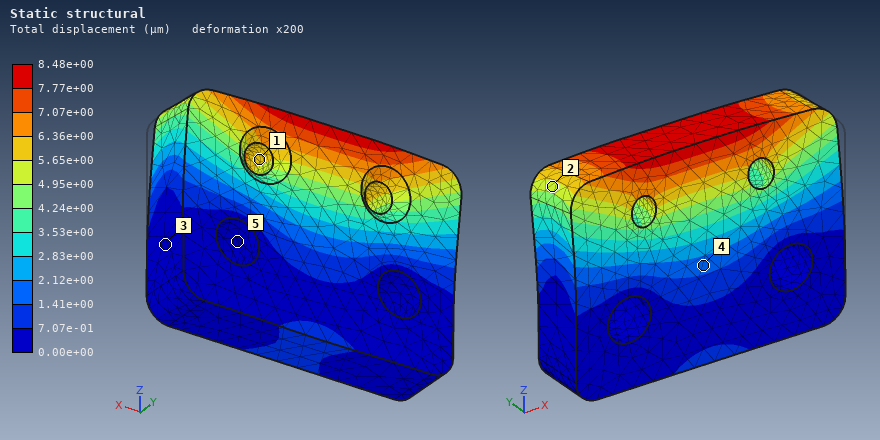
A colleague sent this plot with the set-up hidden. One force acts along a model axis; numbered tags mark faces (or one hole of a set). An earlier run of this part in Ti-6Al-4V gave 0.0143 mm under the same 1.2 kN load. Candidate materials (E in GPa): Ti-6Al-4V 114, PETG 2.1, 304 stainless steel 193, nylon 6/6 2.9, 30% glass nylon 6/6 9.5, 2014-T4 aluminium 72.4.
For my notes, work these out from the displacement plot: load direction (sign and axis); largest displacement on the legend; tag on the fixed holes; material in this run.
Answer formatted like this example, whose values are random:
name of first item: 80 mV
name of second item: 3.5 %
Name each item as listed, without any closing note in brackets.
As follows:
load direction: +Y
largest displacement on the legend: 8.48e+00 µm
tag on the fixed holes: 5
material in this run: 304 stainless steel
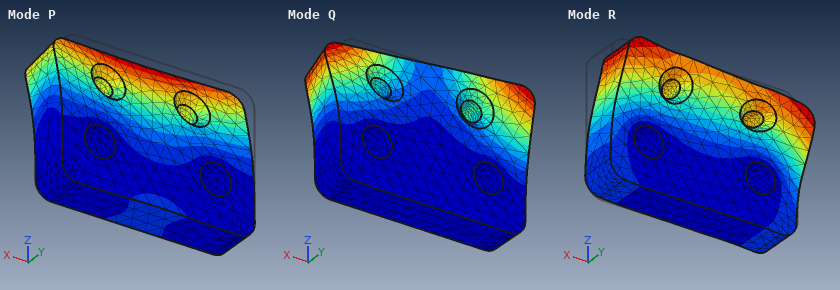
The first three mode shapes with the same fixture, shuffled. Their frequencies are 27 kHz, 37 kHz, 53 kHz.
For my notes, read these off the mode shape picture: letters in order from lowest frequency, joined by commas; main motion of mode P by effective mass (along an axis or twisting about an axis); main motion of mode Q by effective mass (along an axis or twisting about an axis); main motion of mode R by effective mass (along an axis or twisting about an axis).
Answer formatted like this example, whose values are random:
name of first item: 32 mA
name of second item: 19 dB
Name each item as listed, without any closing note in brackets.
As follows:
letters in order from lowest frequency, joined by commas: P, Q, R
main motion of mode P by effective mass: along Y
main motion of mode Q by effective mass: twisting about Z
main motion of mode R by effective mass: along X
